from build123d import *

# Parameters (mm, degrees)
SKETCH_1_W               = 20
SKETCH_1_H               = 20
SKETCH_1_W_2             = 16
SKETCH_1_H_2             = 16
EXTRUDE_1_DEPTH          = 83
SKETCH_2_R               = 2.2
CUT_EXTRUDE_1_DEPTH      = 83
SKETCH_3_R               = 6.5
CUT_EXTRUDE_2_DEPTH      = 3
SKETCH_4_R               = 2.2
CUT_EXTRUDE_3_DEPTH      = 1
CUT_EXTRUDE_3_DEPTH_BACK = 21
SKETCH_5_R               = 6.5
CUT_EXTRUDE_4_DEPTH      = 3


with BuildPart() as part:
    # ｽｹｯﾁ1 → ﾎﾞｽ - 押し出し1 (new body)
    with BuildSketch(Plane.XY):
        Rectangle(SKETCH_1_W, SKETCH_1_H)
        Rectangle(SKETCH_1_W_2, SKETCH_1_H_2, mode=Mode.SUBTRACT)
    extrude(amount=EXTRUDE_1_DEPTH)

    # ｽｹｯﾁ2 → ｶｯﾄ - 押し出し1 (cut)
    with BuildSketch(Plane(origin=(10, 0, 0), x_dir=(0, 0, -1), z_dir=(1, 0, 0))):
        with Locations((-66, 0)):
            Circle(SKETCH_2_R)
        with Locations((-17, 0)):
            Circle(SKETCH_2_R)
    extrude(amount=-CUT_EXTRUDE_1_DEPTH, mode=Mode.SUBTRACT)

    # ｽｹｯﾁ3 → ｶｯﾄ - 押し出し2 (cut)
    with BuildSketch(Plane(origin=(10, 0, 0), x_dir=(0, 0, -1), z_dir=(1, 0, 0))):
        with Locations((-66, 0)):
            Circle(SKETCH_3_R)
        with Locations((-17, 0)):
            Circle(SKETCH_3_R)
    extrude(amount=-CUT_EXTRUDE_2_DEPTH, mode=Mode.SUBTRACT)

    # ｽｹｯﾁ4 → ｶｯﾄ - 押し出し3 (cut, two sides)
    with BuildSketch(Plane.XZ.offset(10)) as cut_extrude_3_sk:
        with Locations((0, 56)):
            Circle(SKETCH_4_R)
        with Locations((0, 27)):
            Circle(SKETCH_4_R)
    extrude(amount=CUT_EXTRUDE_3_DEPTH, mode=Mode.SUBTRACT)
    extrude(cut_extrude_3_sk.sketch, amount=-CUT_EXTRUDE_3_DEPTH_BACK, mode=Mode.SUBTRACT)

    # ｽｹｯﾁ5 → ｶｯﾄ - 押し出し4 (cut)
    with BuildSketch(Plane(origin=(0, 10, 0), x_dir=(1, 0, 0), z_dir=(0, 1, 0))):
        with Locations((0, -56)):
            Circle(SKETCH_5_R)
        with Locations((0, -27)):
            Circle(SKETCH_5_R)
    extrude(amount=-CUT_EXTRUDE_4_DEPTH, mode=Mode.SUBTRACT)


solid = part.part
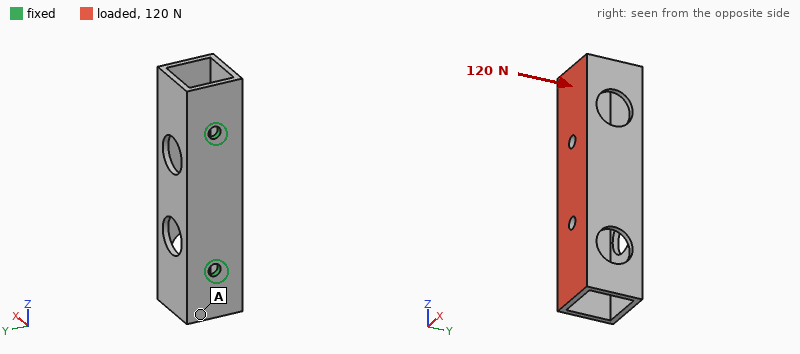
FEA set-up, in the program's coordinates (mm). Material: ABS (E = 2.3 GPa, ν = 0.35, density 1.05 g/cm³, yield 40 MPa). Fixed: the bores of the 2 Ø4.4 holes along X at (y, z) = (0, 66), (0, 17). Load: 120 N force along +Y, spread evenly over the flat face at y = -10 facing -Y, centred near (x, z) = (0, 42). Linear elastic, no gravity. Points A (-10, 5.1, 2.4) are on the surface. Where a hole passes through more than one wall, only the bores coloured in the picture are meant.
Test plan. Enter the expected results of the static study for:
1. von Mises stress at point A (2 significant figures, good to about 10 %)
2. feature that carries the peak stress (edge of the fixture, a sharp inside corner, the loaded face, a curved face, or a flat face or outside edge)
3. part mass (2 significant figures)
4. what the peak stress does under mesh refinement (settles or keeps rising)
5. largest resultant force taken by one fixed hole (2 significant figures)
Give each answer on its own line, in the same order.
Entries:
4.0 MPa
edge of the fixture
11 g
keeps rising
60 N
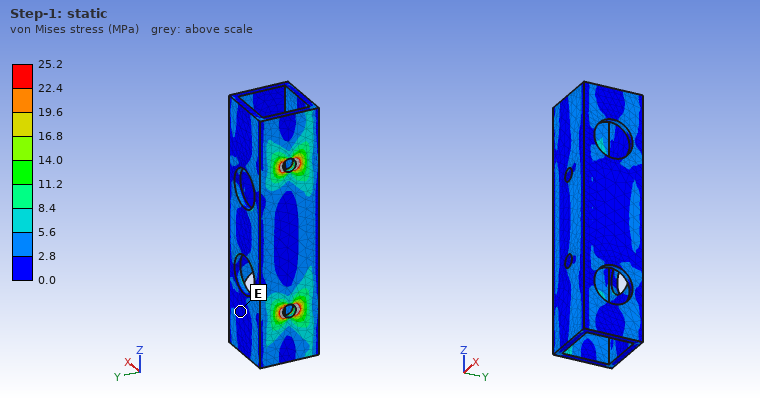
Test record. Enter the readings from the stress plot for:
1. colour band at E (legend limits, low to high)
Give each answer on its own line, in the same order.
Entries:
0.0 to 2.8 MPa
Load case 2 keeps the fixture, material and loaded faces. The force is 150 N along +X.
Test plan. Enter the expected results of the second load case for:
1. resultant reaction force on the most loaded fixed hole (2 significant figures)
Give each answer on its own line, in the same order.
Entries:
75 N
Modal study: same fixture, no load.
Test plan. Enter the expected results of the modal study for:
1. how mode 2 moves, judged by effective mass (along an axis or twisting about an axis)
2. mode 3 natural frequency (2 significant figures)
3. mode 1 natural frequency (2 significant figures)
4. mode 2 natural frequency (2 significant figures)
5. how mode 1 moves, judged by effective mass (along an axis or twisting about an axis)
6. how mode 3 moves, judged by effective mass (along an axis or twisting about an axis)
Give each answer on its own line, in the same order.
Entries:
along Z
1700 Hz
610 Hz
1600 Hz
along Y
along X
